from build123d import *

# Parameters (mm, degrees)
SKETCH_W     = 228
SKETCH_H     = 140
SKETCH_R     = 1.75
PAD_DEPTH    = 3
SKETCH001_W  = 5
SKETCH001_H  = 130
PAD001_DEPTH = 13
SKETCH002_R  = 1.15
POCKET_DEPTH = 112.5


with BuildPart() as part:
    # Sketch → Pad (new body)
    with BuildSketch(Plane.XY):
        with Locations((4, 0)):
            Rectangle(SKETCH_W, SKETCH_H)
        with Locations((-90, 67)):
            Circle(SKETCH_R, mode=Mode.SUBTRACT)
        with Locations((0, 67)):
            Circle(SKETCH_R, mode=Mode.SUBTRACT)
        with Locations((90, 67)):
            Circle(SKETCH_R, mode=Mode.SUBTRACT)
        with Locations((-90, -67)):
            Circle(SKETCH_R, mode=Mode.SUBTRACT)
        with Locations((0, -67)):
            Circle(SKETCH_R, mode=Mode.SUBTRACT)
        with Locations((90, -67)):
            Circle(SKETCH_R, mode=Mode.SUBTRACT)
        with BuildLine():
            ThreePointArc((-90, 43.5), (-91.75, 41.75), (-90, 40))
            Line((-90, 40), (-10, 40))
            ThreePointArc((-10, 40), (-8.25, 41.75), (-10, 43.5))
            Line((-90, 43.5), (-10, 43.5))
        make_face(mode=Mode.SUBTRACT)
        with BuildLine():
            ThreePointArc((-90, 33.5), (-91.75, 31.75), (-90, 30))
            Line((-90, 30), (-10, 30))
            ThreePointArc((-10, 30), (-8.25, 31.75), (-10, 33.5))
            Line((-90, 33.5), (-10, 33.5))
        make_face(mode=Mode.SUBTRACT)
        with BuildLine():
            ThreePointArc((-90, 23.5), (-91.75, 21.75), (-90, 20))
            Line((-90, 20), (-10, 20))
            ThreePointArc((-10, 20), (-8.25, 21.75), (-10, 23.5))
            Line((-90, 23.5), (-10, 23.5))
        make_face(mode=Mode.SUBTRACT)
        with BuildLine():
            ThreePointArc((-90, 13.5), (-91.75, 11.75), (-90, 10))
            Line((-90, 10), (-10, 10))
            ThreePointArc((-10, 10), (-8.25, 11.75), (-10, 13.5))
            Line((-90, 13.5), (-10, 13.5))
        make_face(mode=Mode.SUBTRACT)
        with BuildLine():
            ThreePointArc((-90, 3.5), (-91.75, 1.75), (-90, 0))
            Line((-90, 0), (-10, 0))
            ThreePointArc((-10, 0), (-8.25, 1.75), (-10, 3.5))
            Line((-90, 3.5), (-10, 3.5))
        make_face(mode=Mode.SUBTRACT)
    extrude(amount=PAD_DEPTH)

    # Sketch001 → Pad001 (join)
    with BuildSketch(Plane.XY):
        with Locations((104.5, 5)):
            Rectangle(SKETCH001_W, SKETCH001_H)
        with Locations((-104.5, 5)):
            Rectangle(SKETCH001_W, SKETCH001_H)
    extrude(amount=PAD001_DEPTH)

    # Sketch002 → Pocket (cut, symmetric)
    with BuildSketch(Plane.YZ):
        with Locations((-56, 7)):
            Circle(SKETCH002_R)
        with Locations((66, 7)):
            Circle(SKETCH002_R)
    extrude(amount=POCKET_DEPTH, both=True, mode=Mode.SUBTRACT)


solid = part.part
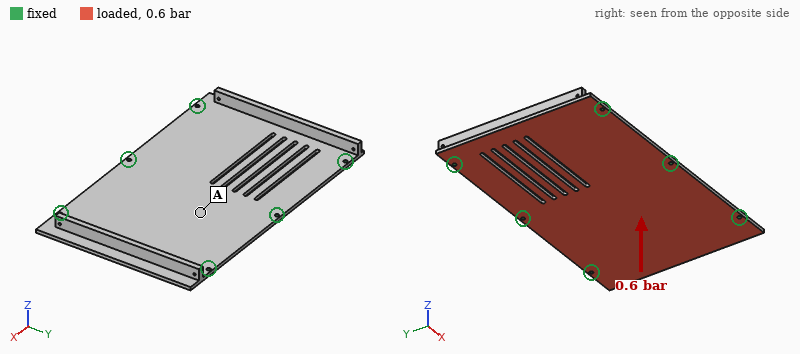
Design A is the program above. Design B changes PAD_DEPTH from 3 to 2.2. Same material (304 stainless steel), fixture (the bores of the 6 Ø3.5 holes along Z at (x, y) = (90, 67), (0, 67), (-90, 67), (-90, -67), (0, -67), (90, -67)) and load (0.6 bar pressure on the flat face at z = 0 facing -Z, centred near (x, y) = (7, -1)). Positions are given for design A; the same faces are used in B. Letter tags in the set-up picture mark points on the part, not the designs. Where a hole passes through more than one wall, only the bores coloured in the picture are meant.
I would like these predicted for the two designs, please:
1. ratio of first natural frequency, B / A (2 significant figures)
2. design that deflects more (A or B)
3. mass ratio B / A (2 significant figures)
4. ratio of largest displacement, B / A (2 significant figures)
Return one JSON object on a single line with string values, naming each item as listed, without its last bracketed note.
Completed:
{"ratio of first natural frequency, B / A": "0.76", "design that deflects more": "B", "mass ratio B / A": "0.78", "ratio of largest displacement, B / A": "2.3"}
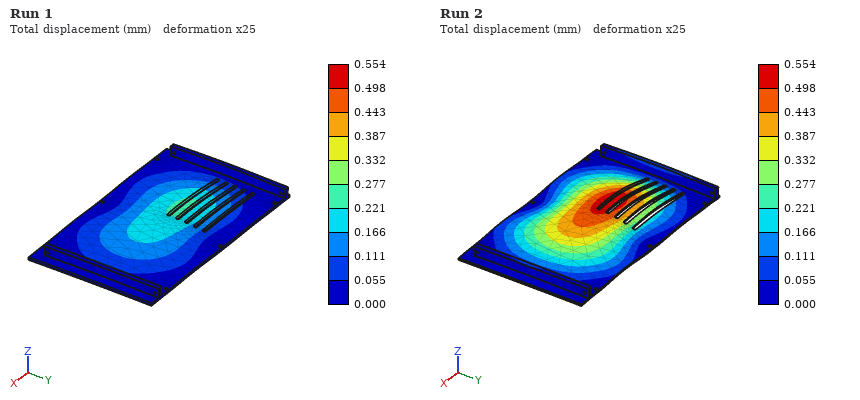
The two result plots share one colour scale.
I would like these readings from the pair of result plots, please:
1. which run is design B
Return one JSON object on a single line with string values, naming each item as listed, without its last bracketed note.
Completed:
{"which run is design B": "Run 2"}
